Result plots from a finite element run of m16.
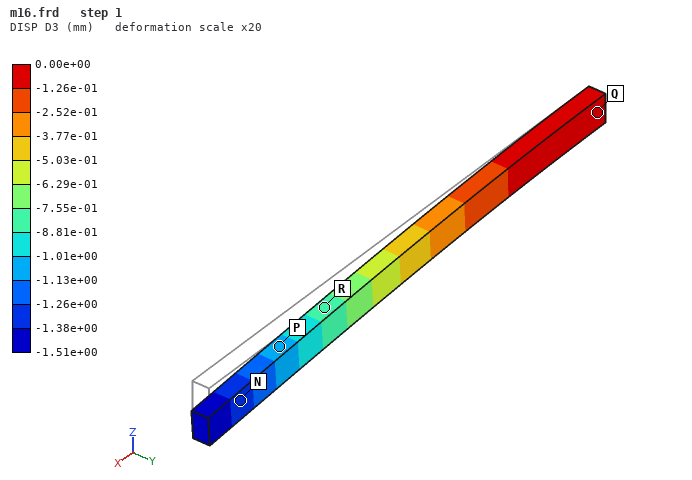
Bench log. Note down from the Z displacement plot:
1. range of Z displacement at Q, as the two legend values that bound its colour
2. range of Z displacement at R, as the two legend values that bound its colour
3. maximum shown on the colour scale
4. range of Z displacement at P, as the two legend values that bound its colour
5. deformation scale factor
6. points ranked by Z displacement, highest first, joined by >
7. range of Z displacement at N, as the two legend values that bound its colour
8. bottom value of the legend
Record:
-1.26e-01 to 0.00e+00 mm
-8.81e-01 to -7.55e-01 mm
0.00e+00 mm
-1.13e+00 to -1.01e+00 mm
20
Q > R > P > N
-1.38e+00 to -1.26e+00 mm
-1.51e+00 mm
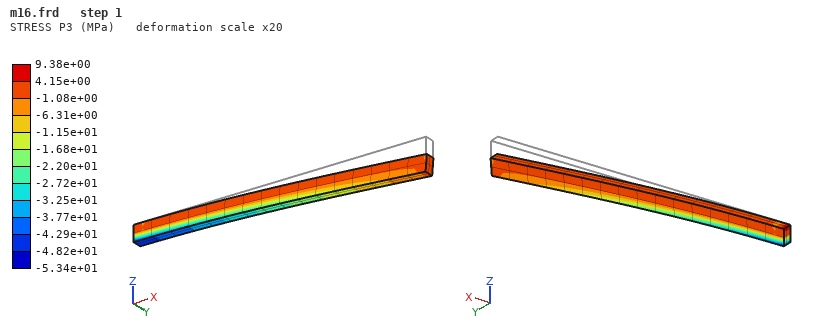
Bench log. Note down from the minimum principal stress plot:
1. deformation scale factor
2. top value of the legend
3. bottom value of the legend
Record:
20
9.38e+00 MPa
-5.34e+01 MPa
